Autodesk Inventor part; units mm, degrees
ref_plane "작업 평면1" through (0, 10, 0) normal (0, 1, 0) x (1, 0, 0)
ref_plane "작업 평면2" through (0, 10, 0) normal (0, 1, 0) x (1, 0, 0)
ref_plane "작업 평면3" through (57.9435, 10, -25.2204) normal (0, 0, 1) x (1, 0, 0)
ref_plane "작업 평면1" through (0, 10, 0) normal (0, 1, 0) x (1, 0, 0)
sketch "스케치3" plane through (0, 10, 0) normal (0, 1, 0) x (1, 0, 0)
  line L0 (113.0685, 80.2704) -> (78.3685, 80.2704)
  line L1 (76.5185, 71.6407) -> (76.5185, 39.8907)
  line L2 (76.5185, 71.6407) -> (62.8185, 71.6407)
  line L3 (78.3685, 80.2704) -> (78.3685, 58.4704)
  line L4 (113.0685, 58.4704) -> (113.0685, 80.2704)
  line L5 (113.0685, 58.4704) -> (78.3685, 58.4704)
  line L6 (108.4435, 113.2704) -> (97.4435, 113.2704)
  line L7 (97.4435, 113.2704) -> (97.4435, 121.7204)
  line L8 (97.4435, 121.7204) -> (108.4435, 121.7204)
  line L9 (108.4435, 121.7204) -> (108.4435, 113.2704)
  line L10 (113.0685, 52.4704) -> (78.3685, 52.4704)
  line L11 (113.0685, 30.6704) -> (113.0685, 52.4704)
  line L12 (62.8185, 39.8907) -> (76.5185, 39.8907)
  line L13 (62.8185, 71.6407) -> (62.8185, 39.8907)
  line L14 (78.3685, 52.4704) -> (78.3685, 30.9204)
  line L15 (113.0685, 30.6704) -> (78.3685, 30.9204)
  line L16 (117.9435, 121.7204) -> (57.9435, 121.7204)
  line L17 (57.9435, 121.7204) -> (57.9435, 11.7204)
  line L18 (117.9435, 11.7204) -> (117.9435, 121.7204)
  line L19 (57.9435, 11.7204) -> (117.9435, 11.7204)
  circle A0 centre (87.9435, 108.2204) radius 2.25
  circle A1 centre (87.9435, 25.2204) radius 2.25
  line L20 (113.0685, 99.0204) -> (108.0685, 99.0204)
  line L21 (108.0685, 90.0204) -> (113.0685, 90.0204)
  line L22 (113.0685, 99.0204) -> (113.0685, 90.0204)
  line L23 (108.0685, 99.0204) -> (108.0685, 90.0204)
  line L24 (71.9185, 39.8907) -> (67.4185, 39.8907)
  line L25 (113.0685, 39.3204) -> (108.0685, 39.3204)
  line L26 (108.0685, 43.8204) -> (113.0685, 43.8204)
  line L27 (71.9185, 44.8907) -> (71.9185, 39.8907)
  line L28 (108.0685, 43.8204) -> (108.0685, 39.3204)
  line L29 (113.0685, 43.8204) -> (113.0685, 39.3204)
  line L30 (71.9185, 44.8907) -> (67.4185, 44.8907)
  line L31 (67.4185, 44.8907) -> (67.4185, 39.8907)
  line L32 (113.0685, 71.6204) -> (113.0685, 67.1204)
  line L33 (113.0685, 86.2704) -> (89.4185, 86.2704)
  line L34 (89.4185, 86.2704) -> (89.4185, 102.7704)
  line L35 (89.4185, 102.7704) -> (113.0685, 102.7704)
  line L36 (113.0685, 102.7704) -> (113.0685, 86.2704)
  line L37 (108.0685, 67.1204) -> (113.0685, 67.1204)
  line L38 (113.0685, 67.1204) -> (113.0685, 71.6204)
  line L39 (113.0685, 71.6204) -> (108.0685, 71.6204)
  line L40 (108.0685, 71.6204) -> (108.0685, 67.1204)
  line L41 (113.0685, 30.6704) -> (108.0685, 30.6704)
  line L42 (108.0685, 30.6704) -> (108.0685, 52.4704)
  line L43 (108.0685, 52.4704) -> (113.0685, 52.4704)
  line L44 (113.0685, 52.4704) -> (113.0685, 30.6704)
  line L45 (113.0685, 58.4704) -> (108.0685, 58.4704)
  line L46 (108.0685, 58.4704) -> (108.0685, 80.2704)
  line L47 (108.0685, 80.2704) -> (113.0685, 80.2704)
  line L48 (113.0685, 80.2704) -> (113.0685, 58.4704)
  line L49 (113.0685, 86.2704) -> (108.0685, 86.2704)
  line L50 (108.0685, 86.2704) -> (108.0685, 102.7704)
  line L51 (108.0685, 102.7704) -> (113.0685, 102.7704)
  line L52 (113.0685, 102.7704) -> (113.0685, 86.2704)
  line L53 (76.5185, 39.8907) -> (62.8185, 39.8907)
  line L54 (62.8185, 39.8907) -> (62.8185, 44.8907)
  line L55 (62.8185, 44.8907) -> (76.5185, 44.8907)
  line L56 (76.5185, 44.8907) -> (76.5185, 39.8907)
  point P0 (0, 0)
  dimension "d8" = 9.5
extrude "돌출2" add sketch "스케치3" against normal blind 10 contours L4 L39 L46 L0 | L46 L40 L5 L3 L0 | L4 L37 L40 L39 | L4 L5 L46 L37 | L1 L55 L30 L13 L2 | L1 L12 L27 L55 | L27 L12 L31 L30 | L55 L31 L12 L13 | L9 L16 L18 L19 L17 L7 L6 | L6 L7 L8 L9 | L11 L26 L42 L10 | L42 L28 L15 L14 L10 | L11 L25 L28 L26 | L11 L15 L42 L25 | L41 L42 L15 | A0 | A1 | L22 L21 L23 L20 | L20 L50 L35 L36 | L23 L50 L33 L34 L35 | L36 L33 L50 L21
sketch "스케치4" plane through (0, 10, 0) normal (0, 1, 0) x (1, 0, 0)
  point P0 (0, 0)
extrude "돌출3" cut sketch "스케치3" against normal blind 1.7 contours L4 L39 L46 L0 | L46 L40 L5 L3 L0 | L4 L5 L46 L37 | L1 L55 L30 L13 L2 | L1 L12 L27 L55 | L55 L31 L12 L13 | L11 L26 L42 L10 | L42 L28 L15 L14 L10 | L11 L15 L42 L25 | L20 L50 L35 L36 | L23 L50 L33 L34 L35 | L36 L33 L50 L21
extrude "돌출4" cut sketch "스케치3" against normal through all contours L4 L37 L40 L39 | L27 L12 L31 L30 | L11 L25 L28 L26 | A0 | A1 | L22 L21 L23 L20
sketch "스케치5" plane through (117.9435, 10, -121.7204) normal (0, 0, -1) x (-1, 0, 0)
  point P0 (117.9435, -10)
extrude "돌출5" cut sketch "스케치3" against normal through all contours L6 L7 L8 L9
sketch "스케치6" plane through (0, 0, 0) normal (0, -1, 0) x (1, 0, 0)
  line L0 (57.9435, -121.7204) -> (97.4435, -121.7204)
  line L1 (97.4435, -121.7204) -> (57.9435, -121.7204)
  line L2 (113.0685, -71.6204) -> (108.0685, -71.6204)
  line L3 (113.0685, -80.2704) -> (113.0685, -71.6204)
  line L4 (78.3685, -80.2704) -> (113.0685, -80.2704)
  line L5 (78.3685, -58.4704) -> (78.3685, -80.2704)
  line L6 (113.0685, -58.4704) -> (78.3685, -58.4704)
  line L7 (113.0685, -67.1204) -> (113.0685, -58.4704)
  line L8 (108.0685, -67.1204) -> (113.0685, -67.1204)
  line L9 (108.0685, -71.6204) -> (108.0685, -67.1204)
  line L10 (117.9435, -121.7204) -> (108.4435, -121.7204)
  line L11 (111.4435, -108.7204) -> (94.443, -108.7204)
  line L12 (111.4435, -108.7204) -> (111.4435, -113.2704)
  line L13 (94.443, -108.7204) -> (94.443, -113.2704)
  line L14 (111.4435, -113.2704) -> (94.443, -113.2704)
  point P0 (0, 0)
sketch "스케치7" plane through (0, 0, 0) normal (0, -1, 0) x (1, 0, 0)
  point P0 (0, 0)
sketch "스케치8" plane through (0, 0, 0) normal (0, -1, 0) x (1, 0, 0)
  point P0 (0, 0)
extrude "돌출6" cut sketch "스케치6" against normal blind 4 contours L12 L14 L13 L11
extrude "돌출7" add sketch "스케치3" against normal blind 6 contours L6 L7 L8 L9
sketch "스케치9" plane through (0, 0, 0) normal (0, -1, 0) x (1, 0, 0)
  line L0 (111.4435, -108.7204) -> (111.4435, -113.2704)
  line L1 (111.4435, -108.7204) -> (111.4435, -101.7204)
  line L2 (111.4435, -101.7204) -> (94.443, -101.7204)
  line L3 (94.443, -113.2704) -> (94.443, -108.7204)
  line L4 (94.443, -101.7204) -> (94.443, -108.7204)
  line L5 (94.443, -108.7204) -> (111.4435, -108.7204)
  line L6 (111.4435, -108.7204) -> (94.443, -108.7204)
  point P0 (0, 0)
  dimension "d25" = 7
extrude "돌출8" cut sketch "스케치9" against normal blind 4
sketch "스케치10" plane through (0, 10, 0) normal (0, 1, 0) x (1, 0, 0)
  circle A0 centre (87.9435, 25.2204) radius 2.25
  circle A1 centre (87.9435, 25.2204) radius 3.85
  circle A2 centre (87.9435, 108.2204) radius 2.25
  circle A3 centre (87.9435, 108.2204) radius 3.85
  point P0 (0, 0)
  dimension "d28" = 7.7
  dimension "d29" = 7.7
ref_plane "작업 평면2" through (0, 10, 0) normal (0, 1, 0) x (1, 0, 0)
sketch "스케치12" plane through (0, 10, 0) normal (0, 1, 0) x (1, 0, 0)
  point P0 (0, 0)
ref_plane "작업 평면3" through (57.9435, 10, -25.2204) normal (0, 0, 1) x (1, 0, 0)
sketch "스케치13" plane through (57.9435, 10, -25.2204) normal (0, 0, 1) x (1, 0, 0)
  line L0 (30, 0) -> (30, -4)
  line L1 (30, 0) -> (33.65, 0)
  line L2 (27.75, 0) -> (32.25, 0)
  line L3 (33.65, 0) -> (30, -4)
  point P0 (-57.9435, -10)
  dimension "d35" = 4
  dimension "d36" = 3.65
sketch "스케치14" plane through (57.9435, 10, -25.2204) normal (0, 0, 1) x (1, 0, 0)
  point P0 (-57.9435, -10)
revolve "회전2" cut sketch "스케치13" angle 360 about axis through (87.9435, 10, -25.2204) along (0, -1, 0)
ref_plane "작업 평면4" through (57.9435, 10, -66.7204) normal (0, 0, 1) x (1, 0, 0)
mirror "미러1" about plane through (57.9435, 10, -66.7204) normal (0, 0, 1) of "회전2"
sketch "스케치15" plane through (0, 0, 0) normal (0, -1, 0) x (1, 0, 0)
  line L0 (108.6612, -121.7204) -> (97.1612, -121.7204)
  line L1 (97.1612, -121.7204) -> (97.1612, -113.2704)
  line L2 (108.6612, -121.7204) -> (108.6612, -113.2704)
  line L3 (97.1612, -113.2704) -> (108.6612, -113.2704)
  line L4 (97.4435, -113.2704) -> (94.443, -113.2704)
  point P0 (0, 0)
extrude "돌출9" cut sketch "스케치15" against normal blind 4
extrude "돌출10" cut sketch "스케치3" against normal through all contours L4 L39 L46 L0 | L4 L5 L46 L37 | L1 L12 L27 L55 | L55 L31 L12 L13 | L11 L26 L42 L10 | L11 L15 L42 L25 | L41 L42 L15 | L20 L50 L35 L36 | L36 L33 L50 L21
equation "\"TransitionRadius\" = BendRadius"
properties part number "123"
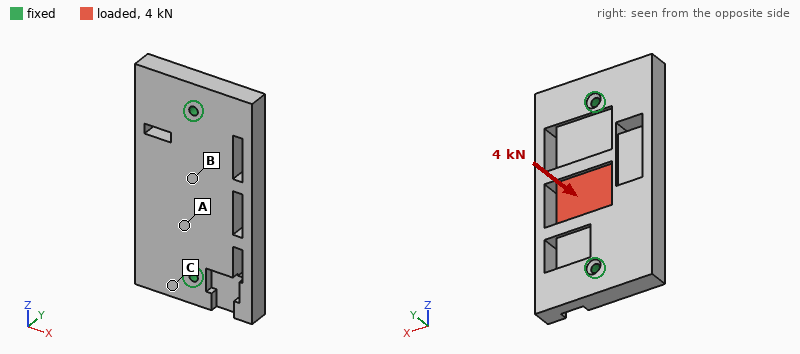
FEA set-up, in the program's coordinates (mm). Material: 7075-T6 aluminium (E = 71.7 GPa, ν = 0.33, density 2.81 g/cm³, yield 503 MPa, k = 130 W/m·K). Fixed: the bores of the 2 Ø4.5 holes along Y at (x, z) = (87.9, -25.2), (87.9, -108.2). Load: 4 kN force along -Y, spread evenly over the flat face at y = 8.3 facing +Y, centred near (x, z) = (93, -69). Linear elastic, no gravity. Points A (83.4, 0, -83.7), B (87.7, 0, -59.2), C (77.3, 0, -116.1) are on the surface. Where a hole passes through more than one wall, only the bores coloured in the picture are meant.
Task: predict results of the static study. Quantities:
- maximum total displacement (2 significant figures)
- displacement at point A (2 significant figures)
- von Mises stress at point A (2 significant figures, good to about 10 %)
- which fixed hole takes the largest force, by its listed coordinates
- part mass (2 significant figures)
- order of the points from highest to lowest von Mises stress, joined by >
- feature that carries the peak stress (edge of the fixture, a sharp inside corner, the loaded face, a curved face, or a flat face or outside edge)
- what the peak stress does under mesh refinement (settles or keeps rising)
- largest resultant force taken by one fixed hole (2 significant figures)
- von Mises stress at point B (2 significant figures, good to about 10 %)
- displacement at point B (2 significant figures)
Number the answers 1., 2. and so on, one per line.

1. 0.13 mm
2. 0.056 mm
3. 28 MPa
4. (87.9, -108.2)
5. 160 g
6. B > A > C
7. edge of the fixture
8. keeps rising
9. 2.2 kN
10. 46 MPa
11. 0.078 mm
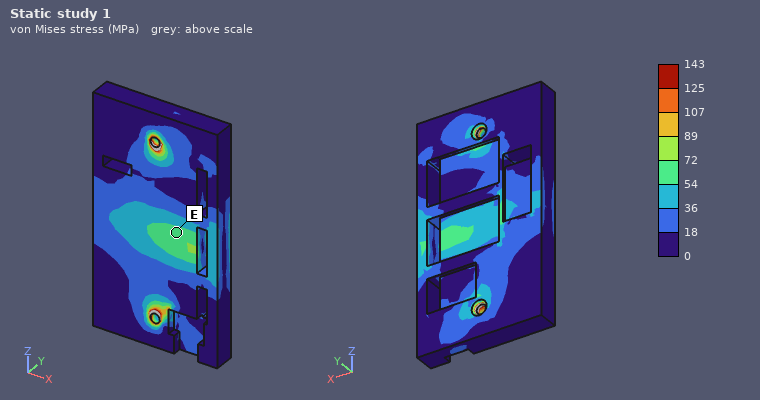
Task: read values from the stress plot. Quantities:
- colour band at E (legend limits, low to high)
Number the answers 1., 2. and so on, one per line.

1. 54 to 72 MPa
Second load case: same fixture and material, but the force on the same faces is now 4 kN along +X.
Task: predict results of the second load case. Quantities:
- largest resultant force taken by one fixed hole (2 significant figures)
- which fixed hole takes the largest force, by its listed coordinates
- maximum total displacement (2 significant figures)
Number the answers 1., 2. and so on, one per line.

1. 2.1 kN
2. (87.9, -108.2)
3. 34 µm
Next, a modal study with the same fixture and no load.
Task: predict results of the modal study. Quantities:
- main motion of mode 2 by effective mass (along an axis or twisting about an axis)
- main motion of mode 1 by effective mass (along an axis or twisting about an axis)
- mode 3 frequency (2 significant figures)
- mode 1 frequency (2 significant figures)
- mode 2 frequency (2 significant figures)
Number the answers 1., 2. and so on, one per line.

1. along Y
2. twisting about Z
3. 6400 Hz
4. 3800 Hz
5. 4400 Hz
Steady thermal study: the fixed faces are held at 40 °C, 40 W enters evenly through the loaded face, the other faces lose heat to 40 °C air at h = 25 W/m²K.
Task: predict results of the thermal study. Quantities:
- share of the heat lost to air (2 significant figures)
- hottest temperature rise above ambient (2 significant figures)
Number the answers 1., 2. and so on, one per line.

1. 8.4 %
2. 19 K
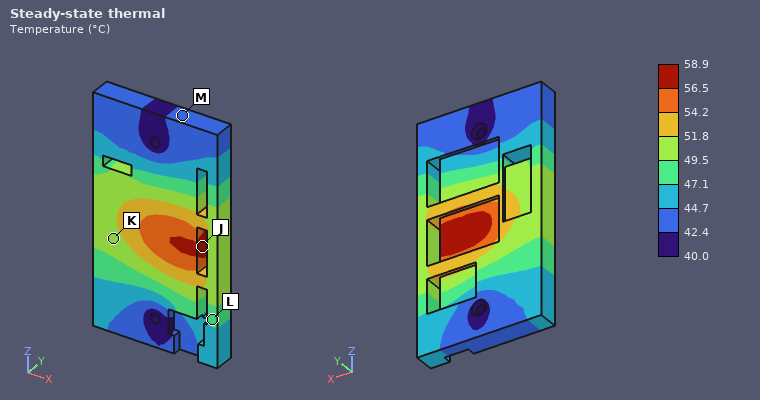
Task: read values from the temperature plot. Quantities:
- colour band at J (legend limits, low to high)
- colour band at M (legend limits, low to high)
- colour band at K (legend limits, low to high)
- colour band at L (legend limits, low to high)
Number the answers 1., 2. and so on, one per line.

1. 56.5 to 58.9 °C
2. 42.4 to 44.7 °C
3. 49.5 to 51.8 °C
4. 47.1 to 49.5 °C
